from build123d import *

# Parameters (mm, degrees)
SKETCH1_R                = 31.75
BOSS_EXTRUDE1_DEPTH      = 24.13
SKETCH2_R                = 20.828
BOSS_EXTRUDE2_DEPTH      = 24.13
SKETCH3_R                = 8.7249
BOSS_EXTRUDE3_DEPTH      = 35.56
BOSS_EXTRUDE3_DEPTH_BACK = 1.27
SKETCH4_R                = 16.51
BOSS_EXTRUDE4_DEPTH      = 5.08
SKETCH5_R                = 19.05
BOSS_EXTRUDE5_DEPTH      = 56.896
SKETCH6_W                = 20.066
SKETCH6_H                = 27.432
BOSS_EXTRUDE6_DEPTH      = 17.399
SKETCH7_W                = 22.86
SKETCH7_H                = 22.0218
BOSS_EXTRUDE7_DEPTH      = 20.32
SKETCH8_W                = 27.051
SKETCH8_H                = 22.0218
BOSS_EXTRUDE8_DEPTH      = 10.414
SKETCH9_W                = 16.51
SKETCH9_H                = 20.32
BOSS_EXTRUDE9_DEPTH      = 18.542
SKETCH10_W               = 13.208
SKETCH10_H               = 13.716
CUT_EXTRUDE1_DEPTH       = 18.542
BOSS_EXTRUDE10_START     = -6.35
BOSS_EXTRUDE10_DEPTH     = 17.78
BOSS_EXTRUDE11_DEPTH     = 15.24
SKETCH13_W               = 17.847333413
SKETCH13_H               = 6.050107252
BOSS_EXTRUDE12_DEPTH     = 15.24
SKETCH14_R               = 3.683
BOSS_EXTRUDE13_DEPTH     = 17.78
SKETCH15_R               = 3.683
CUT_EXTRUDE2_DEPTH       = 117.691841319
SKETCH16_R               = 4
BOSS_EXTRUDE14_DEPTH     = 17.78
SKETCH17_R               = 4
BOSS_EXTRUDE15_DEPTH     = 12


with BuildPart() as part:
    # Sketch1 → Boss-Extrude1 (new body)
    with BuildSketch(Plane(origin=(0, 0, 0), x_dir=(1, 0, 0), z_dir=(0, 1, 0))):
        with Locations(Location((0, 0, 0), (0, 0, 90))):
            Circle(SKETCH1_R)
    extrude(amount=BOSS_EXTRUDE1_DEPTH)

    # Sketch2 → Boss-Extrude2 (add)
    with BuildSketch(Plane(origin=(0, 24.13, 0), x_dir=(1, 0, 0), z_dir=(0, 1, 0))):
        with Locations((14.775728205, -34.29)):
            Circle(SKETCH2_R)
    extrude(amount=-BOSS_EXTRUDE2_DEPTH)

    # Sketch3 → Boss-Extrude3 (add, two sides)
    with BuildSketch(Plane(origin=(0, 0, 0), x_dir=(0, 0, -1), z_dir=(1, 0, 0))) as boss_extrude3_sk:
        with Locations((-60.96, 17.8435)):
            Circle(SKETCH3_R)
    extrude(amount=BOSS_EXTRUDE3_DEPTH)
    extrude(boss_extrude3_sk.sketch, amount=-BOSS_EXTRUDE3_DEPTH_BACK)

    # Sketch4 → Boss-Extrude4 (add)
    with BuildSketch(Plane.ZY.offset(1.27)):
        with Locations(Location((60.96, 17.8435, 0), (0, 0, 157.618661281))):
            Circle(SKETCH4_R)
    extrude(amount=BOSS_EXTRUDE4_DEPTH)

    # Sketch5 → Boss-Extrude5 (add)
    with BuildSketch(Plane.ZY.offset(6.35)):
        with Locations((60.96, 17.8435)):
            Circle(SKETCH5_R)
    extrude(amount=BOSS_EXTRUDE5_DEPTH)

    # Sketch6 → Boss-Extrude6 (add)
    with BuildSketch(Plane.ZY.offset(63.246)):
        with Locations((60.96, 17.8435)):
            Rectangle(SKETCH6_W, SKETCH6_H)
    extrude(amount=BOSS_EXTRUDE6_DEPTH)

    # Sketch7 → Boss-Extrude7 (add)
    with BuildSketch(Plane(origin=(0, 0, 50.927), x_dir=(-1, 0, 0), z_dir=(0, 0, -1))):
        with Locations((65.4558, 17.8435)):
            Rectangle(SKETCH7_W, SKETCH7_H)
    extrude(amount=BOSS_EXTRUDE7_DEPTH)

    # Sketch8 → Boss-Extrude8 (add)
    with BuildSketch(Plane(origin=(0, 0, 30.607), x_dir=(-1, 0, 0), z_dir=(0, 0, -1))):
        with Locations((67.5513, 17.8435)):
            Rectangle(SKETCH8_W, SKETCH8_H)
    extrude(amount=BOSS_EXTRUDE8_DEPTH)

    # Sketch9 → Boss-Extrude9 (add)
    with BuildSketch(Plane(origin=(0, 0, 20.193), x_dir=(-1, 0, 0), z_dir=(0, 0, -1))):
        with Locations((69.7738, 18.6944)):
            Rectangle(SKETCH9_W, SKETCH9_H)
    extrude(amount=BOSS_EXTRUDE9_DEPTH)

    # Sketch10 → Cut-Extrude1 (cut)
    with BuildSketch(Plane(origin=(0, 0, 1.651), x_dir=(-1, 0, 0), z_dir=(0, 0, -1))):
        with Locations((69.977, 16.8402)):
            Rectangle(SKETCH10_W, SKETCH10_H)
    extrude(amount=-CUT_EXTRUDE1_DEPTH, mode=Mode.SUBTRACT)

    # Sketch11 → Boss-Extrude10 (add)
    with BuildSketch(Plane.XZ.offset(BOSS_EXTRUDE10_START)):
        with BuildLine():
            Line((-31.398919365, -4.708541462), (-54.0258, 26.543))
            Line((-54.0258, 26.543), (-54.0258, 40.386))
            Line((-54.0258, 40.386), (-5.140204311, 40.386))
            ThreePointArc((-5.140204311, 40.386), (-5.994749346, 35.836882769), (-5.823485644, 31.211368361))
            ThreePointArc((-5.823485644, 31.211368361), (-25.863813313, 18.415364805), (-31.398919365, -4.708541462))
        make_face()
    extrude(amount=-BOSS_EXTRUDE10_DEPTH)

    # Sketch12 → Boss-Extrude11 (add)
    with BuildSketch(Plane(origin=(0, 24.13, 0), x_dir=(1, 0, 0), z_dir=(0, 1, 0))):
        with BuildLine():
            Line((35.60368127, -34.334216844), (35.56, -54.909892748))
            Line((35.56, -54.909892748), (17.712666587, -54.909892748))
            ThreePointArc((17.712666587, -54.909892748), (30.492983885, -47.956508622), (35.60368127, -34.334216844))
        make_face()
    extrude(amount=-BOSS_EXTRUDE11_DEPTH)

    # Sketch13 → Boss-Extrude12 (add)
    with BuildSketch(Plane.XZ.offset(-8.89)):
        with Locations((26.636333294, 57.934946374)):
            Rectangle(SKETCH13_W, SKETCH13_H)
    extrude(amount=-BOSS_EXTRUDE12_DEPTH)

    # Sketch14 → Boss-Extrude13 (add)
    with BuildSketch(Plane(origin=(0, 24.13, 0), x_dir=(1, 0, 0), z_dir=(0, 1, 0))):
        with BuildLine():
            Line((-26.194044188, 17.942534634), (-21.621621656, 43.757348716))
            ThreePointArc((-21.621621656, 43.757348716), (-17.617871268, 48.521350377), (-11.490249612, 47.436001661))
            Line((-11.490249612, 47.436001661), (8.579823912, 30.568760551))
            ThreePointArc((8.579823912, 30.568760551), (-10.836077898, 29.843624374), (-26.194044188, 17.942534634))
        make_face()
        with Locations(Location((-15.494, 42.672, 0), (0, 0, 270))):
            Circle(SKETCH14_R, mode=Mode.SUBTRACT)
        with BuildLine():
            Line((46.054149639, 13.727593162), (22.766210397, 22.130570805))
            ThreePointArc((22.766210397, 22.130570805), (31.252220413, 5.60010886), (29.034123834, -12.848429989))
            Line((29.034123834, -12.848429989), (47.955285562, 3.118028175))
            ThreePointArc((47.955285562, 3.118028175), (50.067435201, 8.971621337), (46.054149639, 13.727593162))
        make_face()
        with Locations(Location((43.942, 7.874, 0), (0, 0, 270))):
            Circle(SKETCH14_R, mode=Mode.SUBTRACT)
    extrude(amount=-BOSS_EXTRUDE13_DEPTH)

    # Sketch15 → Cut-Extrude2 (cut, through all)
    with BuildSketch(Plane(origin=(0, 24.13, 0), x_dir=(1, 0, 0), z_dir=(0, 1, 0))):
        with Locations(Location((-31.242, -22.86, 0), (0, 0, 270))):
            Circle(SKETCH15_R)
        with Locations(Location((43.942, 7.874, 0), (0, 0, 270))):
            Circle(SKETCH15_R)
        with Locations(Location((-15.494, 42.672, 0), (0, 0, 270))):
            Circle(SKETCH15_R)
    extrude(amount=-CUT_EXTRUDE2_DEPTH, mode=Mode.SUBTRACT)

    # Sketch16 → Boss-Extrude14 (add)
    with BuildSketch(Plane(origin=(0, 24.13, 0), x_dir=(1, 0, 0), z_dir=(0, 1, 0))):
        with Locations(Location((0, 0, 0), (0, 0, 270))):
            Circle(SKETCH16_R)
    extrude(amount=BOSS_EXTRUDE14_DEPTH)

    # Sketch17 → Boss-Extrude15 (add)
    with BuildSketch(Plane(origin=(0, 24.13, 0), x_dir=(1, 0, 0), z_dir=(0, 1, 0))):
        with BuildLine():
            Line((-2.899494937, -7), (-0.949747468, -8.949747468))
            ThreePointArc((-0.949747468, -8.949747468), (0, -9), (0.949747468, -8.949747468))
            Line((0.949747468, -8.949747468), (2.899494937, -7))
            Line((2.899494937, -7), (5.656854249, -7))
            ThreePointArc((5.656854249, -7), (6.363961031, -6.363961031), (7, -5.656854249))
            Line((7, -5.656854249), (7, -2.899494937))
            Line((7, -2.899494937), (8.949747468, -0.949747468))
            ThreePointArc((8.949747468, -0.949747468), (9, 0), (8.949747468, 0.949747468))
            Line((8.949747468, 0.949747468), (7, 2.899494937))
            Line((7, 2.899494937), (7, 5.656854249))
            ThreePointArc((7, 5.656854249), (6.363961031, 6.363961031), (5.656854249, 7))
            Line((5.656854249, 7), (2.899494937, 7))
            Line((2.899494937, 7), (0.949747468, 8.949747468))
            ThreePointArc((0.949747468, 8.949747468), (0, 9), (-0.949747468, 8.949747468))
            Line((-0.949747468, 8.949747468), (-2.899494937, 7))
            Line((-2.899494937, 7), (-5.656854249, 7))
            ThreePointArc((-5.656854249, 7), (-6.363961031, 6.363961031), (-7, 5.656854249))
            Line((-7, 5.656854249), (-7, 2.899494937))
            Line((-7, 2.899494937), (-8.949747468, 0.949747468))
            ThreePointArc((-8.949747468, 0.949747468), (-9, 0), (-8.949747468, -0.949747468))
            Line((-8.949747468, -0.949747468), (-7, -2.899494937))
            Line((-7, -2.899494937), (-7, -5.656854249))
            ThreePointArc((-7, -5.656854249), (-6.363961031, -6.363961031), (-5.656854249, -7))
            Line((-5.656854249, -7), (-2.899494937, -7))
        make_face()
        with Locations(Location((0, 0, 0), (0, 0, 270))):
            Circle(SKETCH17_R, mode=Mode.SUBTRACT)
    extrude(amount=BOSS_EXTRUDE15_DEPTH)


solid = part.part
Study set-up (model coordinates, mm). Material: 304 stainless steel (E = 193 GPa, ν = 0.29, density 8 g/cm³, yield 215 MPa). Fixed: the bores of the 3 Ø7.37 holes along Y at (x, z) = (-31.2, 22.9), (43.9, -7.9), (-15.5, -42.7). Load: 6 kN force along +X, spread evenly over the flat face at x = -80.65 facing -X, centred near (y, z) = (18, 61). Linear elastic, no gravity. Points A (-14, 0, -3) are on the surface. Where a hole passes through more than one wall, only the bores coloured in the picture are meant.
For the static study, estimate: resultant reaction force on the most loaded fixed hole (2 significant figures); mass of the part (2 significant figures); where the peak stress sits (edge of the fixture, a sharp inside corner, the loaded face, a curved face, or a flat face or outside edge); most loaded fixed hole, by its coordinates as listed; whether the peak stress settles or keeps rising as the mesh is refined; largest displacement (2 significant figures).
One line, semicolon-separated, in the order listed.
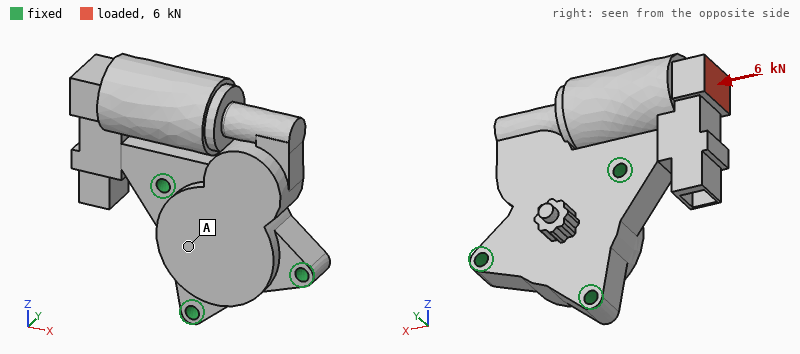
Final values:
6.9 kN; 1.9 kg; edge of the fixture; (-31.2, 22.9); keeps rising; 18 µm
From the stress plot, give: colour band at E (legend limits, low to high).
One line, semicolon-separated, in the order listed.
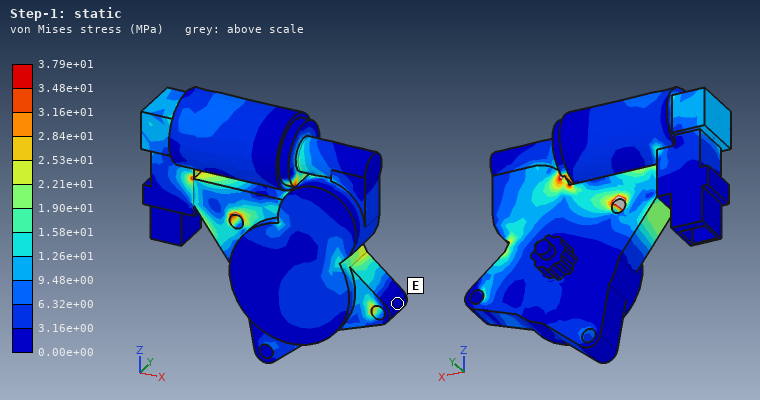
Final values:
0.00e+00 to 3.16e+00 MPa
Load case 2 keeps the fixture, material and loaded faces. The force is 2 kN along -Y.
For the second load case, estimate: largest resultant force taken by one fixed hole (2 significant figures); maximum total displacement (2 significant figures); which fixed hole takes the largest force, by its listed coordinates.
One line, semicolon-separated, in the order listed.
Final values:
2.9 kN; 55 µm; (-31.2, 22.9)
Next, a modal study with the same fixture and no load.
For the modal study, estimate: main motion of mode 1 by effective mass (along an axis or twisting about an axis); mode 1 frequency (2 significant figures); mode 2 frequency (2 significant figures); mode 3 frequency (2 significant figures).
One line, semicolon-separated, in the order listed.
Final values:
along Y; 1900 Hz; 3200 Hz; 3700 Hz
